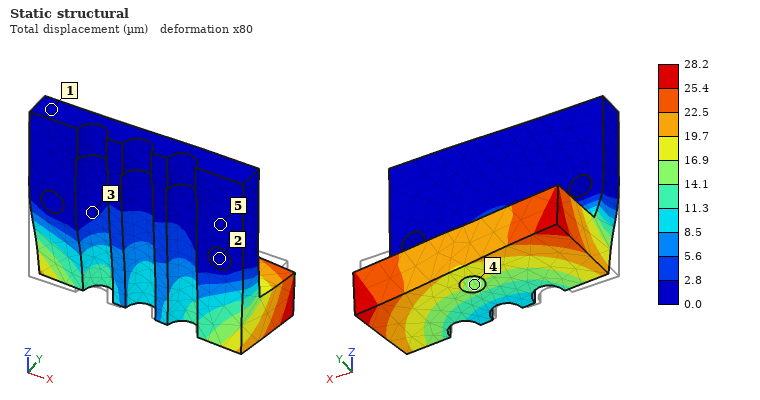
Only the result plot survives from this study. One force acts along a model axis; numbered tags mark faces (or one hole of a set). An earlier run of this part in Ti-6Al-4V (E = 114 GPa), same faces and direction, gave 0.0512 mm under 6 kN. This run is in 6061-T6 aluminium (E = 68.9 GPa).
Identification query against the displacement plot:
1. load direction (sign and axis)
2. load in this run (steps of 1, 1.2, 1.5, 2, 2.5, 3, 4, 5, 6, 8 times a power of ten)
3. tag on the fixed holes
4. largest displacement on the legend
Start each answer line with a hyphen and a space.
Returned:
- +X
- 2 kN
- 2
- 28.2 µm
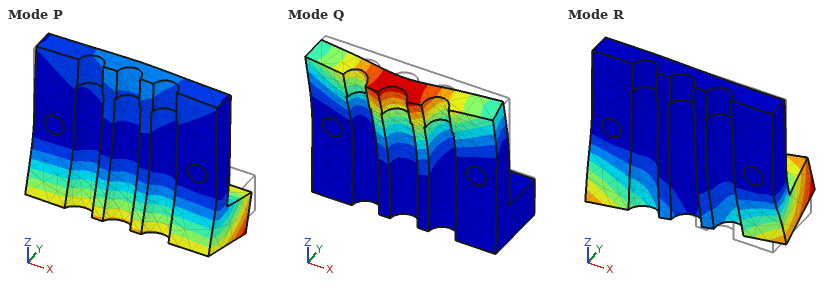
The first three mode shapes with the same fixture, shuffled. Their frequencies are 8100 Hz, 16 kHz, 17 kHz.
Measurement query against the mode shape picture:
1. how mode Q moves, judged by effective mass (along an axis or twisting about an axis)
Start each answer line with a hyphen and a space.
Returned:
- along Y
